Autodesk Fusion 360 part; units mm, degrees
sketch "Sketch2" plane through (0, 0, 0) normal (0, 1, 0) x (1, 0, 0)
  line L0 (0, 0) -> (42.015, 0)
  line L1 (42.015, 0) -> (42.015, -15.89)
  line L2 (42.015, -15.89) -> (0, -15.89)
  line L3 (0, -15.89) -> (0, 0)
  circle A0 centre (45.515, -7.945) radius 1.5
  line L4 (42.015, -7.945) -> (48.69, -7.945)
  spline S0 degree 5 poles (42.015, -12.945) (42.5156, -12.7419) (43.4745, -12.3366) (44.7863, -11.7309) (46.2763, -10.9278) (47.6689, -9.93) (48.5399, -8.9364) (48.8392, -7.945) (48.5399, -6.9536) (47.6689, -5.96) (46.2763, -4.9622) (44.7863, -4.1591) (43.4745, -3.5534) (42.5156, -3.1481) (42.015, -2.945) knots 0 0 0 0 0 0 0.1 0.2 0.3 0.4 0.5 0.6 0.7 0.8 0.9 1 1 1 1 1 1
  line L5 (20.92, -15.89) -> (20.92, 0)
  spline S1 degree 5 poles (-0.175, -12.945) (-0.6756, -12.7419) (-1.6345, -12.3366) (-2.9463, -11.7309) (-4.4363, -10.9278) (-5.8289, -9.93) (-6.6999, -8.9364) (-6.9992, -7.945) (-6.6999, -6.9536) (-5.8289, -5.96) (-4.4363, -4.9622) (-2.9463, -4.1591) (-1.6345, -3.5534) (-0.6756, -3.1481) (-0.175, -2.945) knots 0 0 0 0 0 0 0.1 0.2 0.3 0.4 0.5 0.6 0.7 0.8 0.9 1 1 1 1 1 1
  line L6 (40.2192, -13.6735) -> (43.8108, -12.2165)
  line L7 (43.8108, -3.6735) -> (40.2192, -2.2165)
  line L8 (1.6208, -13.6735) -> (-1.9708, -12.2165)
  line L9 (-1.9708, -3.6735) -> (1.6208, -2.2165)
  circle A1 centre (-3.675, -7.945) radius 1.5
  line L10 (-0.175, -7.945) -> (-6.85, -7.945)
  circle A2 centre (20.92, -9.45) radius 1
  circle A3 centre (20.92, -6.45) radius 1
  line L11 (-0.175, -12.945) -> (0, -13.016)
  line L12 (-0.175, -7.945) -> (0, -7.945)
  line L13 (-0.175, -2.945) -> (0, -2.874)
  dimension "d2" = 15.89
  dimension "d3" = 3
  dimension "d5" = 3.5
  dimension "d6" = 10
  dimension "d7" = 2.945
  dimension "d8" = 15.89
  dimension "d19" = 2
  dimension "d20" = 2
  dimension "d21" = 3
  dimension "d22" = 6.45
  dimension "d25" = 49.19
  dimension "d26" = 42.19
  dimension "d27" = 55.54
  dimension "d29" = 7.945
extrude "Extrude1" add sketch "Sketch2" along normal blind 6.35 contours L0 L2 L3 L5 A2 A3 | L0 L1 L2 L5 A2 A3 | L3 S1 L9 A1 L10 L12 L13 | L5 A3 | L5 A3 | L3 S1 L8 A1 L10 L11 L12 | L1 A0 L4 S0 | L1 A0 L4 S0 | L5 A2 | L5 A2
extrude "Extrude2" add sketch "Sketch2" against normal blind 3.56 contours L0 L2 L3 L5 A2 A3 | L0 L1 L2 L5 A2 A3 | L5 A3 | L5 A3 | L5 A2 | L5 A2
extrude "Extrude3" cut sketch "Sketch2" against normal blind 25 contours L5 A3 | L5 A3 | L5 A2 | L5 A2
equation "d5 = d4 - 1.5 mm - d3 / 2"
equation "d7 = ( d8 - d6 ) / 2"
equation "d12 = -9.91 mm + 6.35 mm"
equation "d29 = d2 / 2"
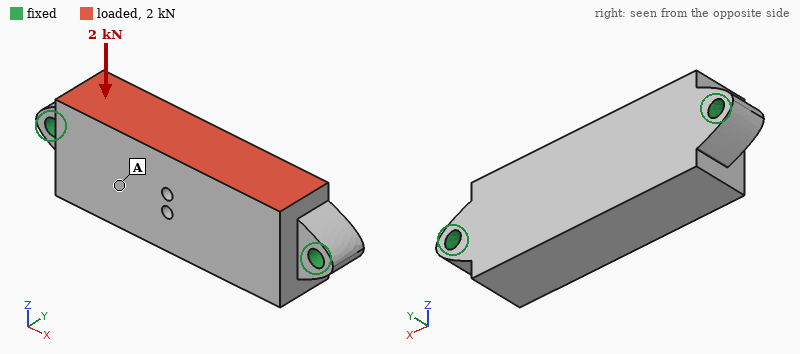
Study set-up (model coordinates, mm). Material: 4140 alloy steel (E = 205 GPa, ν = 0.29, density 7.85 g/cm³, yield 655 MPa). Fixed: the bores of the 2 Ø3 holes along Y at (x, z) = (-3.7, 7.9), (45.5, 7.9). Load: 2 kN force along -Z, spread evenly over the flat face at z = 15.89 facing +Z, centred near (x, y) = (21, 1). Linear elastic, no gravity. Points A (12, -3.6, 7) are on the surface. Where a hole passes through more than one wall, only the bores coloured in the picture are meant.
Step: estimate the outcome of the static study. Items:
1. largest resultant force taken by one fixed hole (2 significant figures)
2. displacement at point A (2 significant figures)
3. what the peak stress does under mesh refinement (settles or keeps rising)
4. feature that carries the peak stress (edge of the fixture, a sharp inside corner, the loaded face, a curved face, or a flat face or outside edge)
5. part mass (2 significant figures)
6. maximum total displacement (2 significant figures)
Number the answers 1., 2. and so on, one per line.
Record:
1. 1.0 kN
2. 6.2 µm
3. keeps rising
4. edge of the fixture
5. 55 g
6. 7.4 µm
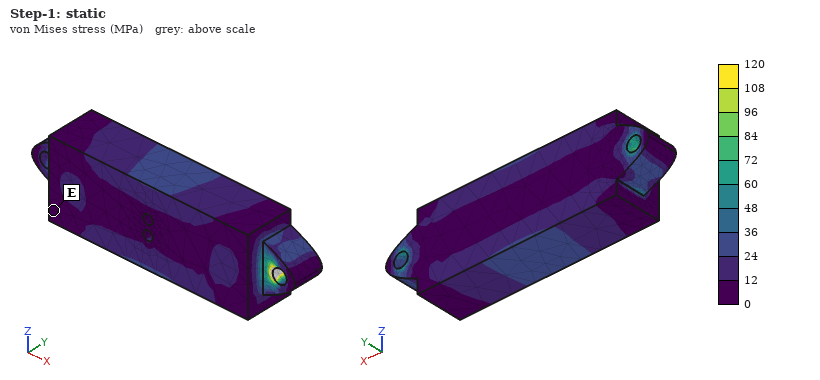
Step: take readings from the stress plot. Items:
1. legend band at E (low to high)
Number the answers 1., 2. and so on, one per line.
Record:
1. 0 to 12 MPa
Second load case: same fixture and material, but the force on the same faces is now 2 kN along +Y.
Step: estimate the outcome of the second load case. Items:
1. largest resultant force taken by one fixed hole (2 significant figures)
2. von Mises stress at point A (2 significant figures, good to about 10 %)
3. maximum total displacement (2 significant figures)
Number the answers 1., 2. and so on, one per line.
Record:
1. 1.2 kN
2. 32 MPa
3. 21 µm
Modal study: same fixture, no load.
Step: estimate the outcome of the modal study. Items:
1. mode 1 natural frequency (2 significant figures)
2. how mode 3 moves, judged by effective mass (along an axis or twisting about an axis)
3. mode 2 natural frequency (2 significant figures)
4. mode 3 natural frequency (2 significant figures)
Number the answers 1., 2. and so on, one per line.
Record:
1. 12 kHz
2. along Z
3. 13 kHz
4. 17 kHz
